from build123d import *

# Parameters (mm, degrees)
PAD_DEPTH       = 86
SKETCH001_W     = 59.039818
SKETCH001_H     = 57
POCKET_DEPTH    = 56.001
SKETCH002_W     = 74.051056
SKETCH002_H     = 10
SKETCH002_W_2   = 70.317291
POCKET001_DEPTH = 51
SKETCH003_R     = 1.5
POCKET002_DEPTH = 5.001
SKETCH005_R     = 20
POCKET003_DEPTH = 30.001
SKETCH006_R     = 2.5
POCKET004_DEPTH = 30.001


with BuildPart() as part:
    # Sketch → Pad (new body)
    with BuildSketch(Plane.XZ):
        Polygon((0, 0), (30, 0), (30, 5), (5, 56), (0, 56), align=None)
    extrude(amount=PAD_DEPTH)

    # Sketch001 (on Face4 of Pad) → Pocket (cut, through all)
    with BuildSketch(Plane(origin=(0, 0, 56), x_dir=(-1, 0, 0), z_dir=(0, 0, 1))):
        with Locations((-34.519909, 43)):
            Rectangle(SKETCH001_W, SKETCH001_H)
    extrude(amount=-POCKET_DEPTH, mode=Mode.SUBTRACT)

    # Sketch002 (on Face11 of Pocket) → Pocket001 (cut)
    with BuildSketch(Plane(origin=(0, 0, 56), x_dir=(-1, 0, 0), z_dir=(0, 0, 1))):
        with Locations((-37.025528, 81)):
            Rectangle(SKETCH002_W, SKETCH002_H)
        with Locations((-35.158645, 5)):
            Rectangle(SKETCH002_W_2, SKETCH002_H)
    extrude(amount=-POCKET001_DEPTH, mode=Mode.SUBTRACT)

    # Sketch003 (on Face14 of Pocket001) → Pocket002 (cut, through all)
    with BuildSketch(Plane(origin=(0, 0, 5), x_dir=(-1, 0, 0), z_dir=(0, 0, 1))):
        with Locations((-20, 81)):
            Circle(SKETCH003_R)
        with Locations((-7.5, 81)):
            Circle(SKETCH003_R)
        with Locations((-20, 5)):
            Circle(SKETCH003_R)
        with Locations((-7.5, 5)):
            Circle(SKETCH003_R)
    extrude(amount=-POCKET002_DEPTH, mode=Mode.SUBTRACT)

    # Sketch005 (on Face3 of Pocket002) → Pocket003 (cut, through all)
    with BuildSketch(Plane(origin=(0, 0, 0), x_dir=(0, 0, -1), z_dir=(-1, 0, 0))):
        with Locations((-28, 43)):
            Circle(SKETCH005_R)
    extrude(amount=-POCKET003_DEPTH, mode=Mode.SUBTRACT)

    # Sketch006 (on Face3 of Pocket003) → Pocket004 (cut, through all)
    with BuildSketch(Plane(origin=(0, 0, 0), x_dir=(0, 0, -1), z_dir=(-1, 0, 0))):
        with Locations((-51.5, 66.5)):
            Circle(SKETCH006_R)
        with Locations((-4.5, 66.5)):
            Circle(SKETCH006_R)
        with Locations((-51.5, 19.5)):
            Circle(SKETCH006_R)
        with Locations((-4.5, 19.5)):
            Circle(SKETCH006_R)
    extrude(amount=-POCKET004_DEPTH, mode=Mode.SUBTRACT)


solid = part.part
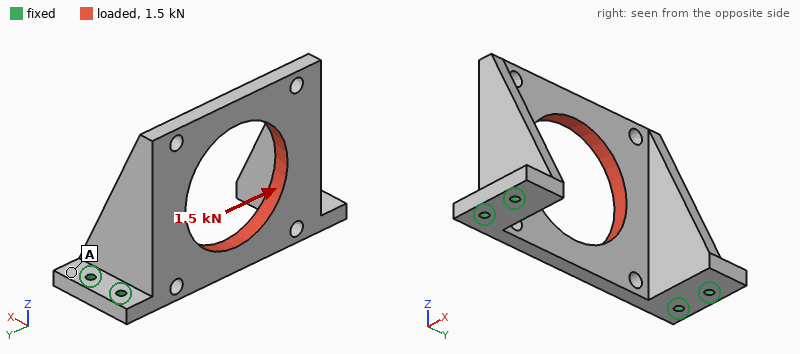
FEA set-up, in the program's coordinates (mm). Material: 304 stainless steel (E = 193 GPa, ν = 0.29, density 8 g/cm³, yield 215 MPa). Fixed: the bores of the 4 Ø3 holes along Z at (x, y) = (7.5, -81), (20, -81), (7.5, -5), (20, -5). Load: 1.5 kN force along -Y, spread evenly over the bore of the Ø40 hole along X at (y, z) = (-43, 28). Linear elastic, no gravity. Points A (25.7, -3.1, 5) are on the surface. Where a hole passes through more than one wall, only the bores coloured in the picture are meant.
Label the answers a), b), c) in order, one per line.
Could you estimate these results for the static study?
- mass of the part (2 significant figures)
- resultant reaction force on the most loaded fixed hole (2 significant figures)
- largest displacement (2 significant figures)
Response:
a) 170 g
b) 1.0 kN
c) 21 µm
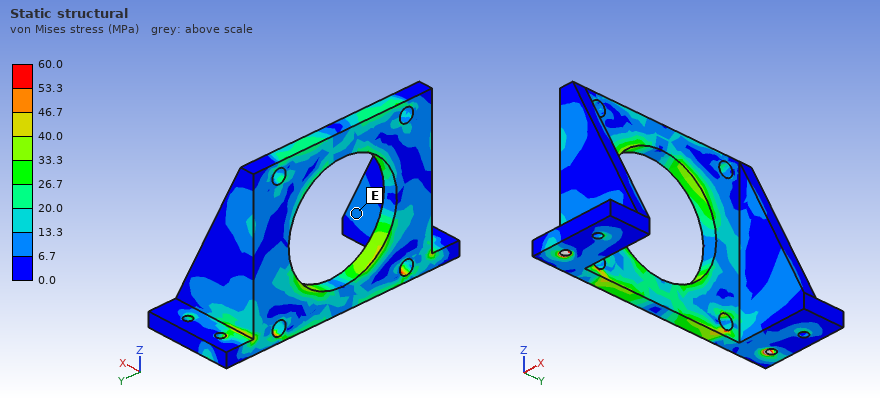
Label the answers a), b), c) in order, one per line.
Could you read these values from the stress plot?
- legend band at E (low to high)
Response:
a) 6.7 to 13.3 MPa
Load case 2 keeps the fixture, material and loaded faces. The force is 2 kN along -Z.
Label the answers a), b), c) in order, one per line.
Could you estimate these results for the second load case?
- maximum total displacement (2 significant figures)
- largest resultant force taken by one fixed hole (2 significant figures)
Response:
a) 27 µm
b) 1.2 kN
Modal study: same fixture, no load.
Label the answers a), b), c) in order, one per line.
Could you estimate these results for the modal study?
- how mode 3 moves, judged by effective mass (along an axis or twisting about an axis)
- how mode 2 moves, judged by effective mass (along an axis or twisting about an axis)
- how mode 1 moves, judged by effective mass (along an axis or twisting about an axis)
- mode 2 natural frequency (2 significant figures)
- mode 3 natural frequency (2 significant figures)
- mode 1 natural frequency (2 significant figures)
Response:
a) along Y
b) along Y
c) along X
d) 3700 Hz
e) 5200 Hz
f) 2700 Hz
